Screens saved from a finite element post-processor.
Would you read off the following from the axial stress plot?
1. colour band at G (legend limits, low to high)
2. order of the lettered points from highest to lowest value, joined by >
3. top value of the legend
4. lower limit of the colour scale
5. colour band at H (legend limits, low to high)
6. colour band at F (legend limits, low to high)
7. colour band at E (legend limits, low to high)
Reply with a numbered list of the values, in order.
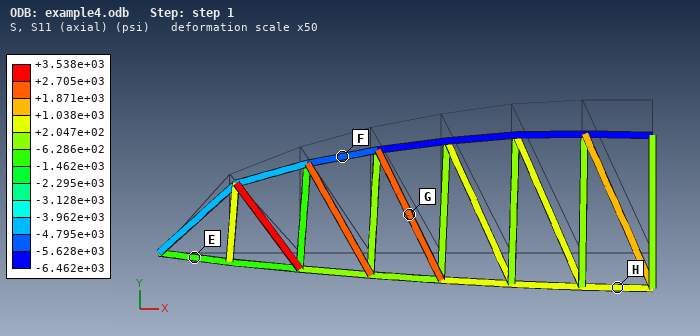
1. +1.871e+03 to +2.705e+03 psi
2. G > H > E > F
3. +3.538e+03 psi
4. -6.462e+03 psi
5. +2.047e+02 to +1.038e+03 psi
6. -5.628e+03 to -4.795e+03 psi
7. -1.462e+03 to -6.286e+02 psi
